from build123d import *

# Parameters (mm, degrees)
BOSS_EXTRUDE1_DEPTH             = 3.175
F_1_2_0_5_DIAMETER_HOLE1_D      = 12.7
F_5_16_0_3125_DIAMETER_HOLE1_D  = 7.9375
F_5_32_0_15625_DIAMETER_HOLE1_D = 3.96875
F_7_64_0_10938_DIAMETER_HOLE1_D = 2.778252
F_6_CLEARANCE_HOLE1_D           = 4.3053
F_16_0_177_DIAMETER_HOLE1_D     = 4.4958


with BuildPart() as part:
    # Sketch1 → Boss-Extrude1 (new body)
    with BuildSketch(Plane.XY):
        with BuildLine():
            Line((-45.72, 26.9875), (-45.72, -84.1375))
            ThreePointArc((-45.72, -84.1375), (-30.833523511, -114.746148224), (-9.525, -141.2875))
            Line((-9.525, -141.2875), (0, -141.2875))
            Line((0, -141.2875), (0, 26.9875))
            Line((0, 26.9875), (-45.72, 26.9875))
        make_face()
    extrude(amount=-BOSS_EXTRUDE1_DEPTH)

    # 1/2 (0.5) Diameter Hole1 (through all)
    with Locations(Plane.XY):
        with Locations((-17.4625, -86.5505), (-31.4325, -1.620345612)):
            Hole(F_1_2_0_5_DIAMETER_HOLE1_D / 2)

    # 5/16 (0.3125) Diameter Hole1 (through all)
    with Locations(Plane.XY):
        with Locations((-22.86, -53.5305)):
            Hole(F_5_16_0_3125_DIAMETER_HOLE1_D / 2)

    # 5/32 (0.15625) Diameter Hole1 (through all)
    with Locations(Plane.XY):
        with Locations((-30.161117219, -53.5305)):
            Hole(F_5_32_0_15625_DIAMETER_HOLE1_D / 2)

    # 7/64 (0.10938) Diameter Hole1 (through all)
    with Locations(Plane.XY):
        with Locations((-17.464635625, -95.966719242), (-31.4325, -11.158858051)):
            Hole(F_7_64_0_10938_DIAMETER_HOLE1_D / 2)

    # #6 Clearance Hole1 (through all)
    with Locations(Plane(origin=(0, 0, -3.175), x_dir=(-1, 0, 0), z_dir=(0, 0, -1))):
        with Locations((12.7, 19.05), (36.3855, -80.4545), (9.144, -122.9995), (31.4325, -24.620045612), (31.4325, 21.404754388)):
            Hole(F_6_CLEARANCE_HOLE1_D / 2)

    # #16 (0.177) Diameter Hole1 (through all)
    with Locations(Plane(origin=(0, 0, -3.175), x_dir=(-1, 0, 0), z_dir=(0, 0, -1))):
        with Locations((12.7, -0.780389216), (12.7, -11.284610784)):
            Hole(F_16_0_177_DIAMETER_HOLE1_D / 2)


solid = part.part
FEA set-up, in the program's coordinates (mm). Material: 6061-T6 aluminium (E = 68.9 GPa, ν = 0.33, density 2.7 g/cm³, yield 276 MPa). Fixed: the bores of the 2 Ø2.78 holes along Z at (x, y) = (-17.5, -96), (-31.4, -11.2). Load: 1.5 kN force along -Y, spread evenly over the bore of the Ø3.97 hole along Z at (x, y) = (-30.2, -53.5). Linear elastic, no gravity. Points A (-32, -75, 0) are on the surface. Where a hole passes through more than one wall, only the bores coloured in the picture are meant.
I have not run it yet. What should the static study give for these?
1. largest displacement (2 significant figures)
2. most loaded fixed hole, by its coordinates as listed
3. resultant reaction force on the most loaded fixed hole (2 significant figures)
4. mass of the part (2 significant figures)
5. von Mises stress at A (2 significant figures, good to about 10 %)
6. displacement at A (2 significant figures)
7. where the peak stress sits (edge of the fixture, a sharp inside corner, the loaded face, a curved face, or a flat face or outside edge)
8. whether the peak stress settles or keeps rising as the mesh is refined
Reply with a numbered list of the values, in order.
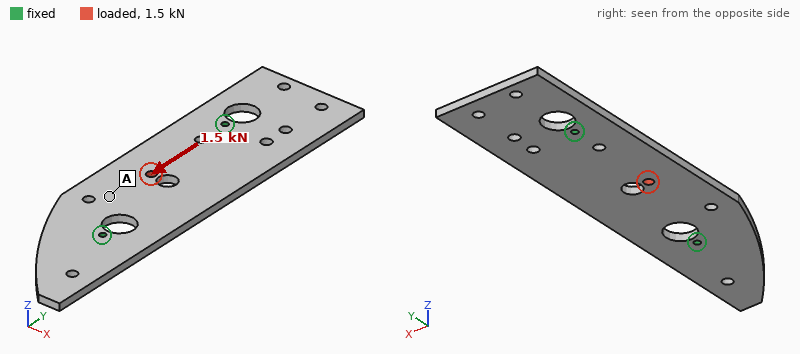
1. 12 µm
2. (-31.4, -11.2)
3. 860 N
4. 55 g
5. 9.7 MPa
6. 7.8 µm
7. edge of the fixture
8. keeps rising
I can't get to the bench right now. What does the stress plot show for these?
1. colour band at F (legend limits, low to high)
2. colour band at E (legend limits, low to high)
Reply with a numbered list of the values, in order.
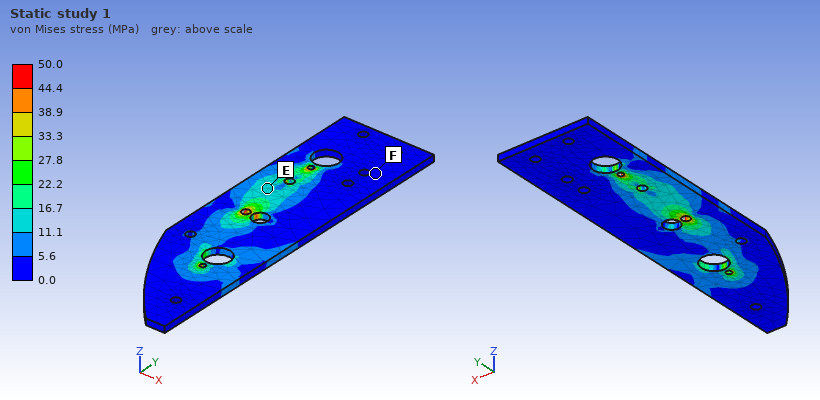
1. 0.0 to 5.6 MPa
2. 11.1 to 16.7 MPa
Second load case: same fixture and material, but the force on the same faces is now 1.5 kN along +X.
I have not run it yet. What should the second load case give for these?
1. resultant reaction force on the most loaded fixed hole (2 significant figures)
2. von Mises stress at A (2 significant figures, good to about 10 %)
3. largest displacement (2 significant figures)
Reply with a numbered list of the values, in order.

1. 760 N
2. 10 MPa
3. 32 µm
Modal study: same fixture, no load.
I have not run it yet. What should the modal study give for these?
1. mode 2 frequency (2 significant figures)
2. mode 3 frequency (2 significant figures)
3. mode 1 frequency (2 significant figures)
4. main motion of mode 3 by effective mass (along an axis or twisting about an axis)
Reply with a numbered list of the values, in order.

1. 1400 Hz
2. 1600 Hz
3. 1100 Hz
4. along Z
